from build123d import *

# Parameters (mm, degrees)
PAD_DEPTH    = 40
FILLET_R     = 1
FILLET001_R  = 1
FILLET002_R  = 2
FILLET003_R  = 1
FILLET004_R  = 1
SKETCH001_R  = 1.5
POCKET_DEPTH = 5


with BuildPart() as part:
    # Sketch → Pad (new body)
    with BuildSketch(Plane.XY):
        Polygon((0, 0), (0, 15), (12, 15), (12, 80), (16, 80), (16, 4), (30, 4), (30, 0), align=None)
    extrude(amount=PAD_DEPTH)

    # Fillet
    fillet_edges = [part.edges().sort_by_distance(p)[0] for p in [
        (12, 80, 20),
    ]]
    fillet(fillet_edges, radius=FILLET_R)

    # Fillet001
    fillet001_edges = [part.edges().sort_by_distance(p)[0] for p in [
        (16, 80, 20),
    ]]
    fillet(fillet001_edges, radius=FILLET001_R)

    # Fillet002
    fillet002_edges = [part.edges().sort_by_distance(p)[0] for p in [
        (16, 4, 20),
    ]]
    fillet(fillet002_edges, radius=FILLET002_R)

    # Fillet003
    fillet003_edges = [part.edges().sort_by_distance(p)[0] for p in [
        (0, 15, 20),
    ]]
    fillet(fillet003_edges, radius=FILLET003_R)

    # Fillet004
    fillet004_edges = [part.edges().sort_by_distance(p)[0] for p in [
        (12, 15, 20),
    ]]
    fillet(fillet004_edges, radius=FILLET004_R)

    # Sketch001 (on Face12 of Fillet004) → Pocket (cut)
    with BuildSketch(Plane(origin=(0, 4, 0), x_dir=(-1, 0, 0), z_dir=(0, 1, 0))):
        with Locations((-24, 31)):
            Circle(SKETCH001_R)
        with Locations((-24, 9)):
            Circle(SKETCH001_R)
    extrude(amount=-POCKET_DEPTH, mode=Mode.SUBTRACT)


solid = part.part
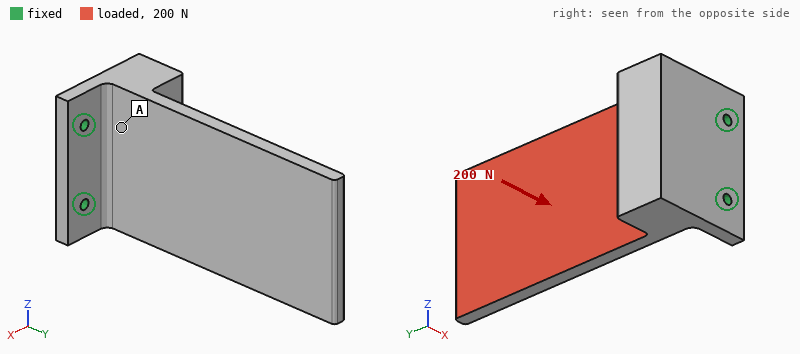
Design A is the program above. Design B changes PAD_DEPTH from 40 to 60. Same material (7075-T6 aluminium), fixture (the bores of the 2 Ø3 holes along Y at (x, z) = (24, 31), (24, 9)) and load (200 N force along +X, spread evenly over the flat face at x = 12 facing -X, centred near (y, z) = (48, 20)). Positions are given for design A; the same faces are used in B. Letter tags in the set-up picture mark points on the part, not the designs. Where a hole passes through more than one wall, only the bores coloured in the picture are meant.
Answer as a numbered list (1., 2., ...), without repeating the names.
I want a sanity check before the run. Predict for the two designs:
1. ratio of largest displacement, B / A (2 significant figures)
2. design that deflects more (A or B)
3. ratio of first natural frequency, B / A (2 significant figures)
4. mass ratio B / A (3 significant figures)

1. 0.77
2. A
3. 0.93
4. 1.50
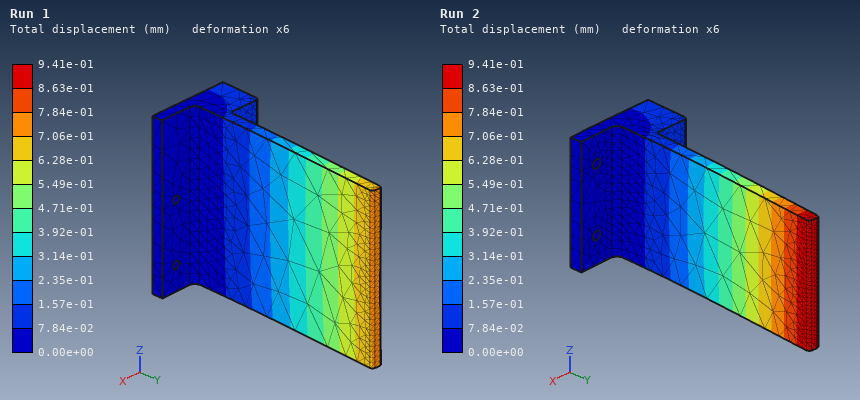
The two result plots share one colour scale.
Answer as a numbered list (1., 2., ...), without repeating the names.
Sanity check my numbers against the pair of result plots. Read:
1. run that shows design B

1. Run 1
